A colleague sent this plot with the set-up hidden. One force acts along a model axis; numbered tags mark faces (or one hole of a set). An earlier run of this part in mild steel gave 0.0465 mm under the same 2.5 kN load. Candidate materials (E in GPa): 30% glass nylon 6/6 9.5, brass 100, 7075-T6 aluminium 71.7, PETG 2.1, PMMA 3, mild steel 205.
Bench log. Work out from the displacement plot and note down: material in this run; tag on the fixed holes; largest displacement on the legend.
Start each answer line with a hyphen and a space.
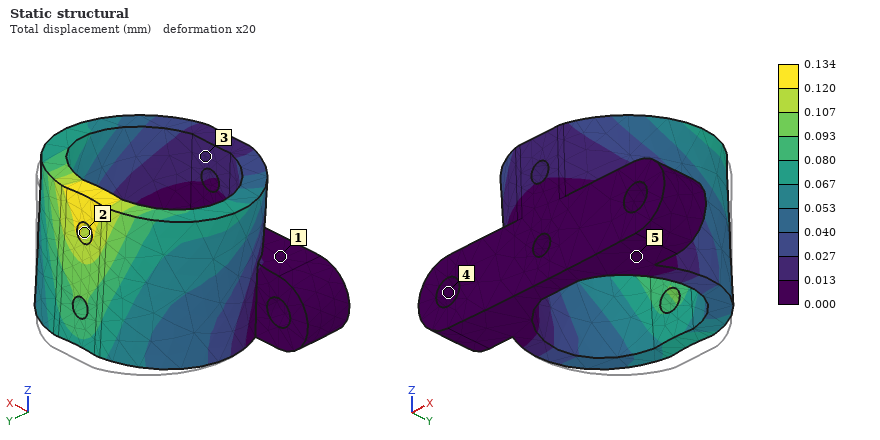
- 7075-T6 aluminium
- 4
- 0.134 mm
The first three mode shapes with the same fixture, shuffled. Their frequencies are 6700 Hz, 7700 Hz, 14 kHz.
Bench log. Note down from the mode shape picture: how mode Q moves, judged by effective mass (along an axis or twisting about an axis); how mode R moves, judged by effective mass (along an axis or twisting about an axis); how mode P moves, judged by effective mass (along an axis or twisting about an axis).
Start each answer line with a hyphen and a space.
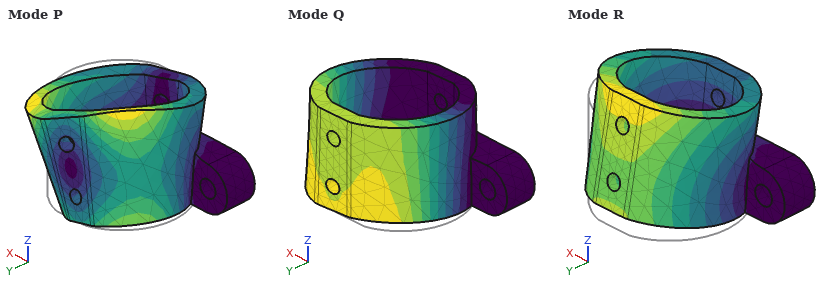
- along X
- along Z
- twisting about Y
